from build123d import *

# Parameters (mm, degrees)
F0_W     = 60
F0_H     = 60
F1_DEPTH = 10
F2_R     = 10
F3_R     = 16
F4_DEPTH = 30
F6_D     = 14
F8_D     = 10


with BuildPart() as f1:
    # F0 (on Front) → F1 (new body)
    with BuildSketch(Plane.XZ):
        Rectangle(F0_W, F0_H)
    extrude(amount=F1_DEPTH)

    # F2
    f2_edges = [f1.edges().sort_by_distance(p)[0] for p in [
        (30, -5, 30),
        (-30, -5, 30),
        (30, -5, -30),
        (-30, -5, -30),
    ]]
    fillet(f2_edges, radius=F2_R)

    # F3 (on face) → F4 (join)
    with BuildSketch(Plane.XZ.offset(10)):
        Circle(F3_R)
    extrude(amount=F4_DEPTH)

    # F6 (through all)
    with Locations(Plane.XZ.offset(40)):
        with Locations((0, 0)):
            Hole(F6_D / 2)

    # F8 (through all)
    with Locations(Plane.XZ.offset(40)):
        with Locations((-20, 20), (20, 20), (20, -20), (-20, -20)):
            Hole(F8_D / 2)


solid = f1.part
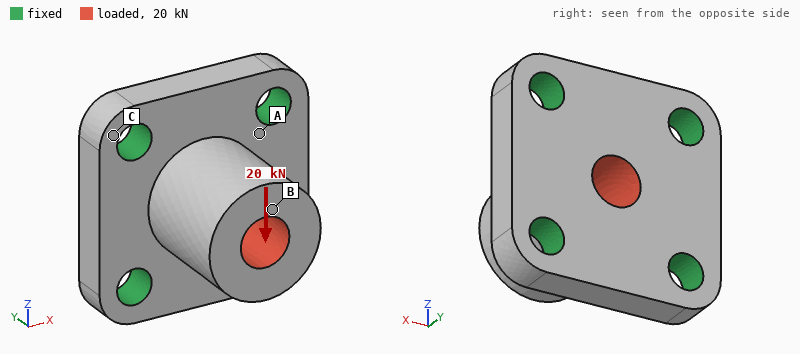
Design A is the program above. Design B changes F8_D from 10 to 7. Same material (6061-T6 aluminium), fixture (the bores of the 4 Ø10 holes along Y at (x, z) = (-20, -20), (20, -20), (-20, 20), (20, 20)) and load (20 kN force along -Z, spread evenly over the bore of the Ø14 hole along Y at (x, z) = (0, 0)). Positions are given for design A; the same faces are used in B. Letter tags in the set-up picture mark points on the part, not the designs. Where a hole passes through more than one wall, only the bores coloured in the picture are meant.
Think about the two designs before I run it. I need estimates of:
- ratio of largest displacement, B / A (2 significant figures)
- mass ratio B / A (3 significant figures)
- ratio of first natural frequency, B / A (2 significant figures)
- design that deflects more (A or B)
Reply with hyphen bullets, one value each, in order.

- 1.1
- 1.03
- 0.94
- B
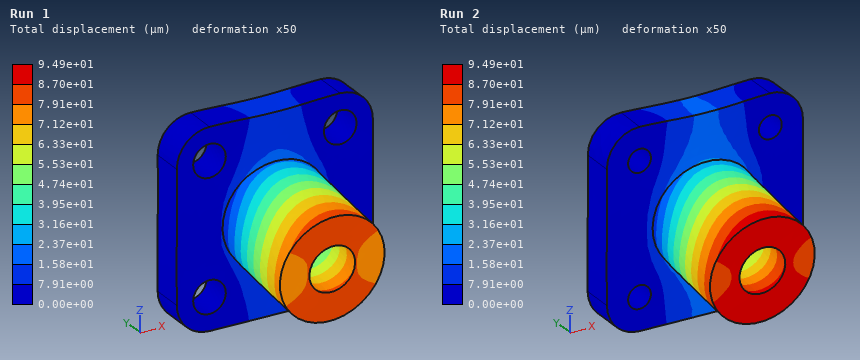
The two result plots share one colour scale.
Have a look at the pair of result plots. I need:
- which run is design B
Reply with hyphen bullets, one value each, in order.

- Run 2
